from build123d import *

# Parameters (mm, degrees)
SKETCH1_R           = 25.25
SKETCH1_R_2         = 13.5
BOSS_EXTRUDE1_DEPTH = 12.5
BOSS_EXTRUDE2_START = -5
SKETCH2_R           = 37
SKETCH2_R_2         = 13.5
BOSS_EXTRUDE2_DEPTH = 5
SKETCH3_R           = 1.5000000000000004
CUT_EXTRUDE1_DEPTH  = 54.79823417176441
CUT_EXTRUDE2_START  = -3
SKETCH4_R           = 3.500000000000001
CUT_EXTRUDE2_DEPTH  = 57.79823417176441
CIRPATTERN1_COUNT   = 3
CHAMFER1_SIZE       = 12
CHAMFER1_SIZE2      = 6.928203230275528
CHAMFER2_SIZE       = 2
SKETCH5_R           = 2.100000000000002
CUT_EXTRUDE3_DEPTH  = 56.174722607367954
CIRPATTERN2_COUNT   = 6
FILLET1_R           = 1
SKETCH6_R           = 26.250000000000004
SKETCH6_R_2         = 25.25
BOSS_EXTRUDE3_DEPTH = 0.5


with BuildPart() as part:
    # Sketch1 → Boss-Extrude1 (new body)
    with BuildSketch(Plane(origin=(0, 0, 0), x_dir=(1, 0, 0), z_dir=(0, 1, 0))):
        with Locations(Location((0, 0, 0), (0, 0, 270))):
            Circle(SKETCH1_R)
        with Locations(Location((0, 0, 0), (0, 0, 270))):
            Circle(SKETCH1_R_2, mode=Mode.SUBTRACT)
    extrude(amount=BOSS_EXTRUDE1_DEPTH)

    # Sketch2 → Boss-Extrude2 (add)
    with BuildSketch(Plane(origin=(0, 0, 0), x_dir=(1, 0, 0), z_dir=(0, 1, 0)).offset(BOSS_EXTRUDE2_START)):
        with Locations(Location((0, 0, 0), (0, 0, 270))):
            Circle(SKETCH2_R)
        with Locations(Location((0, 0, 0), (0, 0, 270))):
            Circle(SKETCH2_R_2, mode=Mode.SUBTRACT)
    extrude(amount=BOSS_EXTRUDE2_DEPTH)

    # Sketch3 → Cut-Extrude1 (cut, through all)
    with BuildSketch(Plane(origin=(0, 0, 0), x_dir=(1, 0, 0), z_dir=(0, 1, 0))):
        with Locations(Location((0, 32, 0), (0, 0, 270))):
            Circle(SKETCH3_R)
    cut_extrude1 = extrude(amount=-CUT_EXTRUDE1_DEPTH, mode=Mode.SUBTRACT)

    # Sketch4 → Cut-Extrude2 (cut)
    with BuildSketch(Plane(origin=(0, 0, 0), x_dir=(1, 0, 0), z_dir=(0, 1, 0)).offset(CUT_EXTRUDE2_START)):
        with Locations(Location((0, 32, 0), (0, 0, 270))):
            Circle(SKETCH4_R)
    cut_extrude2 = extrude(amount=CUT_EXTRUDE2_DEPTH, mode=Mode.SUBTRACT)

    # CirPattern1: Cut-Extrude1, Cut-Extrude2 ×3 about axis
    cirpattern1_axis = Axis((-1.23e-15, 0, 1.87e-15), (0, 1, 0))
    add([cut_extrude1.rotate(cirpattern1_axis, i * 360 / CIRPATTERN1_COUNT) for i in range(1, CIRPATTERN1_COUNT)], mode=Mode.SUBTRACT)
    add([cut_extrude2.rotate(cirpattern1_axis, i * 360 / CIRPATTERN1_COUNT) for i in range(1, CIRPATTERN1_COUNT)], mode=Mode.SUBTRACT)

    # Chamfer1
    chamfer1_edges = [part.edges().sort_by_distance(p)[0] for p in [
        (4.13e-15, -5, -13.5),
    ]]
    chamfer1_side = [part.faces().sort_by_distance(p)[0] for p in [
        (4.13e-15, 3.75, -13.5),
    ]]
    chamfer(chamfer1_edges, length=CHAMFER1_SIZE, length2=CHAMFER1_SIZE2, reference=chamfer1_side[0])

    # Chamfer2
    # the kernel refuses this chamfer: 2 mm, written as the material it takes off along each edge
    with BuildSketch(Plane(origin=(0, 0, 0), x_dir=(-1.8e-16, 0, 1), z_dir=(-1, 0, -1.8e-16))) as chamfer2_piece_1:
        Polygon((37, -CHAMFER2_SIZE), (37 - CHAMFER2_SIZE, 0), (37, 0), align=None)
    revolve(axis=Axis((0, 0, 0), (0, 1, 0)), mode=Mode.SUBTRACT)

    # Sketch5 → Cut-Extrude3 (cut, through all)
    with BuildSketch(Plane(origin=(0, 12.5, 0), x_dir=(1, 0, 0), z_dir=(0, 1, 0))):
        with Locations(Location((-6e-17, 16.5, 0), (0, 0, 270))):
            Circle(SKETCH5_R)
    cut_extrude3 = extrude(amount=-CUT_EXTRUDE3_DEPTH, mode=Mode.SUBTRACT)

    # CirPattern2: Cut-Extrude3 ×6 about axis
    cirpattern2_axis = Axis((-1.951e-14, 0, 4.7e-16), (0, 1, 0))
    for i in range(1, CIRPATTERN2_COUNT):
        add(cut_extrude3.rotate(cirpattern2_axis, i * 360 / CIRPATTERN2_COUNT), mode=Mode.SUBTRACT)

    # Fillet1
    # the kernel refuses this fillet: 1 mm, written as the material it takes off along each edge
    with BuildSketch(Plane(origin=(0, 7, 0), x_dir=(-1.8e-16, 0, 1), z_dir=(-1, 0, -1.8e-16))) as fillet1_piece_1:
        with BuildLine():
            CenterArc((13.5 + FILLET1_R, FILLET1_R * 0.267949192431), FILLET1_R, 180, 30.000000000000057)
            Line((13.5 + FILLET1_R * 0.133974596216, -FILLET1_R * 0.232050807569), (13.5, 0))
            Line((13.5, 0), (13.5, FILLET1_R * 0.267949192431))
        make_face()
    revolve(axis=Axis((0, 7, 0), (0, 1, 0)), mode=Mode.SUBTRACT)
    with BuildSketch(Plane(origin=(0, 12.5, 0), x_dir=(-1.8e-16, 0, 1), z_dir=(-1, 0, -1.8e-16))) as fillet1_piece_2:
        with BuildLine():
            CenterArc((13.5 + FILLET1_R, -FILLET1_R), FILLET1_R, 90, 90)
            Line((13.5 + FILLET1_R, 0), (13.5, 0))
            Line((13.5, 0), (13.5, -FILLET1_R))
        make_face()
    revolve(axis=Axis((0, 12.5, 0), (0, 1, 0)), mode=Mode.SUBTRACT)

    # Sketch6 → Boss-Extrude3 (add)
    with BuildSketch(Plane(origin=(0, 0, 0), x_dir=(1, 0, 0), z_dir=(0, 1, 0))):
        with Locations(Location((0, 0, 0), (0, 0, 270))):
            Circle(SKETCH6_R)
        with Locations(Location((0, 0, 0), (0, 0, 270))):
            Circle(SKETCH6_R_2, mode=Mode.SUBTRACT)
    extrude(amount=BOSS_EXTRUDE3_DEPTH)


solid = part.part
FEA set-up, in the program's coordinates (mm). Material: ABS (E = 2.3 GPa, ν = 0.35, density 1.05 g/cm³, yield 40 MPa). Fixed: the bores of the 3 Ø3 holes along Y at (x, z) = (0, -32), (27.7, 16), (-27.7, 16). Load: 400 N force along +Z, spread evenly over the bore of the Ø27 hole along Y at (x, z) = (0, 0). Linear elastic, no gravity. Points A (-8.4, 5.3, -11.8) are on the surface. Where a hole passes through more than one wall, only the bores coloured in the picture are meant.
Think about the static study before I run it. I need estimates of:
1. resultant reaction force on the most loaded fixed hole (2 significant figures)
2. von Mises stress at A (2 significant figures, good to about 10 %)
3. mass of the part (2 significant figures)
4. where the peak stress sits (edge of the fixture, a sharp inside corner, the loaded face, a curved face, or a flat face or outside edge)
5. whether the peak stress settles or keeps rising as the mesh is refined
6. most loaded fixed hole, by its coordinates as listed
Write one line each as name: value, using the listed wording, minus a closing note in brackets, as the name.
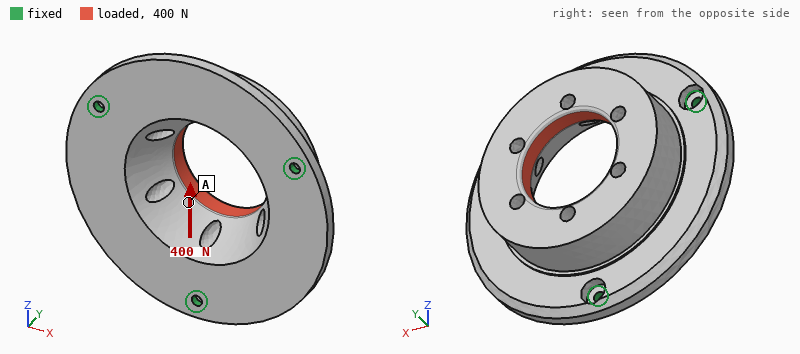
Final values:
resultant reaction force on the most loaded fixed hole: 200 N
von Mises stress at A: 1.2 MPa
mass of the part: 32 g
where the peak stress sits: edge of the fixture
whether the peak stress settles or keeps rising as the mesh is refined: keeps rising
most loaded fixed hole, by its coordinates as listed: (0, -32)
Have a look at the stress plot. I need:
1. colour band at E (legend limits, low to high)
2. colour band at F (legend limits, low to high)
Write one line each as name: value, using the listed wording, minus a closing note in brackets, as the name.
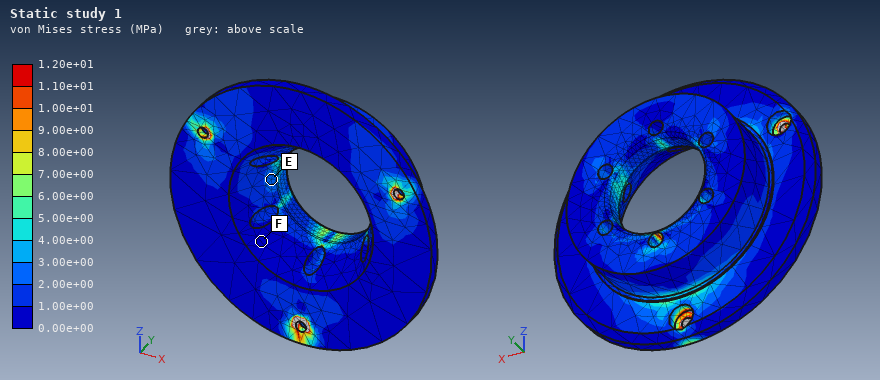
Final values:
colour band at E: 2.00e+00 to 3.00e+00 MPa
colour band at F: 0.00e+00 to 1.00e+00 MPa
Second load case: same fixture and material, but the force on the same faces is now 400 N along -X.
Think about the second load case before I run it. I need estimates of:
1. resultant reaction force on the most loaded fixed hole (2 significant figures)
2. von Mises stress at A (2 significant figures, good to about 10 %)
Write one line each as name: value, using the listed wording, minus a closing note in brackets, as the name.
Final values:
resultant reaction force on the most loaded fixed hole: 180 N
von Mises stress at A: 2.0 MPa
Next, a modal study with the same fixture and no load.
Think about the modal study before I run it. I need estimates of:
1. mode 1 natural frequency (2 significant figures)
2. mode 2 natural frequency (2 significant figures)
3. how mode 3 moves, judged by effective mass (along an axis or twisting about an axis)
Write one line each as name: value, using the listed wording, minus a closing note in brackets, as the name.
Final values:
mode 1 natural frequency: 1900 Hz
mode 2 natural frequency: 1900 Hz
how mode 3 moves, judged by effective mass: along Y
